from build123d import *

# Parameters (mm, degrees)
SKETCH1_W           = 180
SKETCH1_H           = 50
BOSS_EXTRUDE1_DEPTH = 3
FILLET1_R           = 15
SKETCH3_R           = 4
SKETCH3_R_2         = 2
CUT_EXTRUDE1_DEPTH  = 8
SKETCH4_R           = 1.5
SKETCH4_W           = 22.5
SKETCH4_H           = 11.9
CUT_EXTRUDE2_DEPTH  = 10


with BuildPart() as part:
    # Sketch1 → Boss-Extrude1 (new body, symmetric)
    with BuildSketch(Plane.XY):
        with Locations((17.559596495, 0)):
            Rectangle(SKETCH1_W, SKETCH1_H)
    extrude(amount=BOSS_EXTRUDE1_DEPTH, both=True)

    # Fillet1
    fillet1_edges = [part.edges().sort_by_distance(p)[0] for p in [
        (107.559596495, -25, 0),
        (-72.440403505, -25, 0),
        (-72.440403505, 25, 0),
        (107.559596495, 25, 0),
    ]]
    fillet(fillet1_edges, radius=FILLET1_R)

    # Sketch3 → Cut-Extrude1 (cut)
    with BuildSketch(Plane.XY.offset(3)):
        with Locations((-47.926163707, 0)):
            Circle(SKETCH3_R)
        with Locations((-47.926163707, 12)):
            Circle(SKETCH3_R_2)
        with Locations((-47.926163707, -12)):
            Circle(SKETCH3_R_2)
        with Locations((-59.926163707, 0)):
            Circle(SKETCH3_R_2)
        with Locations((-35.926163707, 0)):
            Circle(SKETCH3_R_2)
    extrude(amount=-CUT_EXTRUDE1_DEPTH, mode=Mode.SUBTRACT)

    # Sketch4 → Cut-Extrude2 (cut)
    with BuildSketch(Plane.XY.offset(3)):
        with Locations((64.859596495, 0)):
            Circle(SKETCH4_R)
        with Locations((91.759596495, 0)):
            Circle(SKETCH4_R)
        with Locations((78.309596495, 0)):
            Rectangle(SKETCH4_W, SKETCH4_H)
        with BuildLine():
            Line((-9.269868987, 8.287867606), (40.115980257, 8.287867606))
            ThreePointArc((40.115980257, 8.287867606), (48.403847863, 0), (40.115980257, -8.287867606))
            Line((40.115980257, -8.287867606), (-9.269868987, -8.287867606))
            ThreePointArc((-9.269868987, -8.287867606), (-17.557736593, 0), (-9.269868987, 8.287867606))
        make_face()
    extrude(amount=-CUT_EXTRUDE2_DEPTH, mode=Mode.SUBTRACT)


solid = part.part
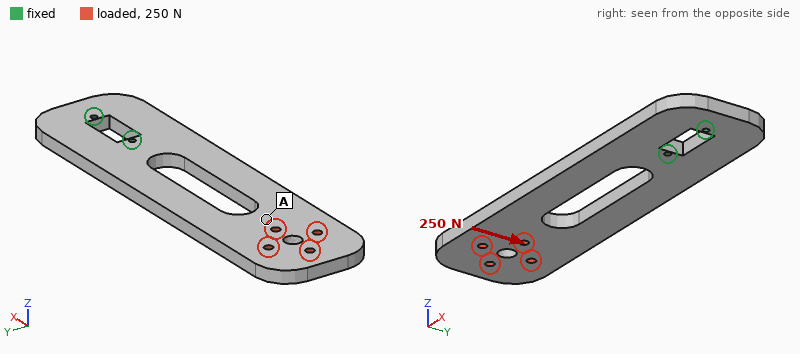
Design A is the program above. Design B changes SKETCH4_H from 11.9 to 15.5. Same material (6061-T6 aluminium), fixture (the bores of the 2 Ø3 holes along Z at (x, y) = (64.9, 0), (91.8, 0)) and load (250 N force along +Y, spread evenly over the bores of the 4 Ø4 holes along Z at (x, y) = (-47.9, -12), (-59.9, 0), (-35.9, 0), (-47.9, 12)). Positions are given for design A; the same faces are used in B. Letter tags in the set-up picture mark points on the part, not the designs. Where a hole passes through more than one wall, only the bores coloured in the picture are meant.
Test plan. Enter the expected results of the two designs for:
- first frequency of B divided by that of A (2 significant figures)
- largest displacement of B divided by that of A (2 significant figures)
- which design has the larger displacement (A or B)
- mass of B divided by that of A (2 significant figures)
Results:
1.00
1.1
B
0.99
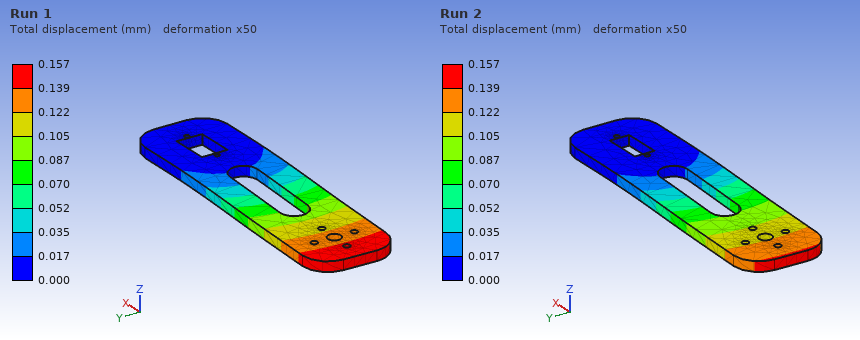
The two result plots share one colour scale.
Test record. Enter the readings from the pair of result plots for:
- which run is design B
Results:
Run 1
